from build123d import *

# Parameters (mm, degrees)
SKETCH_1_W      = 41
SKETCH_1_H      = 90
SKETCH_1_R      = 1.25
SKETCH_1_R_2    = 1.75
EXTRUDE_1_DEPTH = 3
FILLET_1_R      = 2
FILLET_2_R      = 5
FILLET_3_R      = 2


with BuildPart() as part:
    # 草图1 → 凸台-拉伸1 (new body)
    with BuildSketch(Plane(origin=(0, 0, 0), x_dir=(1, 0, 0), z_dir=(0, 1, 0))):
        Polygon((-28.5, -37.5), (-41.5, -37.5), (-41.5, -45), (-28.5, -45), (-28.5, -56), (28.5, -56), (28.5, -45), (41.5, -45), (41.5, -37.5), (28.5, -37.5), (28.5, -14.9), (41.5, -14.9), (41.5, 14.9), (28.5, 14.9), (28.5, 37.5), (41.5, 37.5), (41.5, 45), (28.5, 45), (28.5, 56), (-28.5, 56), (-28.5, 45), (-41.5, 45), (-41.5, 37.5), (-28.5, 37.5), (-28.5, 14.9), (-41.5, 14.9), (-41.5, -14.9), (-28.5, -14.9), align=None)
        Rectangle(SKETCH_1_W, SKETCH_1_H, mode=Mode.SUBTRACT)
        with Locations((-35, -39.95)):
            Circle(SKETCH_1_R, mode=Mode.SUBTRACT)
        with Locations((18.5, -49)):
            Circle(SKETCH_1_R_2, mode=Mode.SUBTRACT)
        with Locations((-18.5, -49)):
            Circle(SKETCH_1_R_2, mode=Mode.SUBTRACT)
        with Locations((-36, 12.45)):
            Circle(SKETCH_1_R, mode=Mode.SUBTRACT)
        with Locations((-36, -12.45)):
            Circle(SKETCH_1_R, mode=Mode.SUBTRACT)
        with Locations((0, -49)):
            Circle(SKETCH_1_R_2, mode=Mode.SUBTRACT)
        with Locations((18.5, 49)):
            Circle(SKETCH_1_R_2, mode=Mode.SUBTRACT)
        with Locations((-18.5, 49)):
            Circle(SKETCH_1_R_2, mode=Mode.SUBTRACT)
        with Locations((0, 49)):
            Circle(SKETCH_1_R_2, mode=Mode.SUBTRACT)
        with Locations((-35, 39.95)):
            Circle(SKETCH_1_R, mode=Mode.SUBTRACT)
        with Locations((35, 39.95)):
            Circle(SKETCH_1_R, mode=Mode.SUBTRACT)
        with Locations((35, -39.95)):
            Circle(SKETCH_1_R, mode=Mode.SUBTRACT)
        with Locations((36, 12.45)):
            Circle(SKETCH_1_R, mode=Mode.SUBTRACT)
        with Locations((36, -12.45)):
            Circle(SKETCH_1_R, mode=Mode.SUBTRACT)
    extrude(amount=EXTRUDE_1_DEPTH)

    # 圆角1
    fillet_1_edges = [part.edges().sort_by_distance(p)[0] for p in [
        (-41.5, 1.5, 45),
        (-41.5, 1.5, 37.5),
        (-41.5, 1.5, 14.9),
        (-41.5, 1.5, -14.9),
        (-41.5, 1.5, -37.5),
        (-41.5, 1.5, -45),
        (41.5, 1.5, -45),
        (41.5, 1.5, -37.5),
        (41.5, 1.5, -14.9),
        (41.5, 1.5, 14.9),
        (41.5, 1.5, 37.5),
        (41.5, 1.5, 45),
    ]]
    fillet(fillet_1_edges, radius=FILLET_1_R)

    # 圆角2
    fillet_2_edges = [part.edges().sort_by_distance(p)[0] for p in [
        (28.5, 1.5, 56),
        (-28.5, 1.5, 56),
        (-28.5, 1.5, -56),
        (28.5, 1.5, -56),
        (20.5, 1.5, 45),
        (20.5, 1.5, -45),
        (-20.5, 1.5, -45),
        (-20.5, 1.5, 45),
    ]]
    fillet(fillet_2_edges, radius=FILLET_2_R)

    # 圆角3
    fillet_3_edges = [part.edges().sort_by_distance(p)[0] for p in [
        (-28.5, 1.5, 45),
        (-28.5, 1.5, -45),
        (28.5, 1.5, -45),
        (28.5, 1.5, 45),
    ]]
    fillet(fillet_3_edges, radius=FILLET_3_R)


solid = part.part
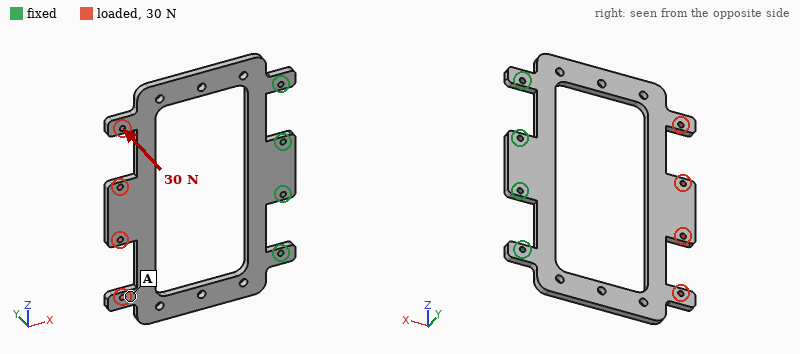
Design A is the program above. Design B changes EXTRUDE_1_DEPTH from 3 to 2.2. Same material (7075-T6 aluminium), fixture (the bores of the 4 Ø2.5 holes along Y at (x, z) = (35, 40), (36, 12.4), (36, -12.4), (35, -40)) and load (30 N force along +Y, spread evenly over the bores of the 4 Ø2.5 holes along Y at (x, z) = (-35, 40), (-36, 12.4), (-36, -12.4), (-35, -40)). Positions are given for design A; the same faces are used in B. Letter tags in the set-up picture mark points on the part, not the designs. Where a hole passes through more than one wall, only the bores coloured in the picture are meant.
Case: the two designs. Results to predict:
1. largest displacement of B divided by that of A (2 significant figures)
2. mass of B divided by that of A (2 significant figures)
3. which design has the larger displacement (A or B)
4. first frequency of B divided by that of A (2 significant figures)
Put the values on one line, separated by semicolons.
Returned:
2.5; 0.73; B; 0.74
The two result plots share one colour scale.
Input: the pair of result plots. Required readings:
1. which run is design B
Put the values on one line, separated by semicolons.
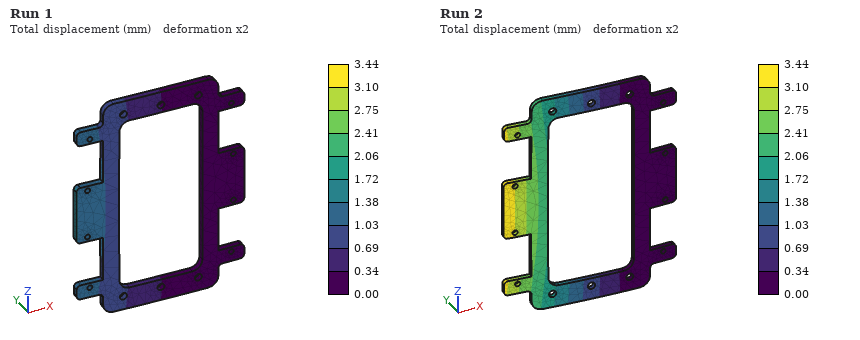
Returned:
Run 2
